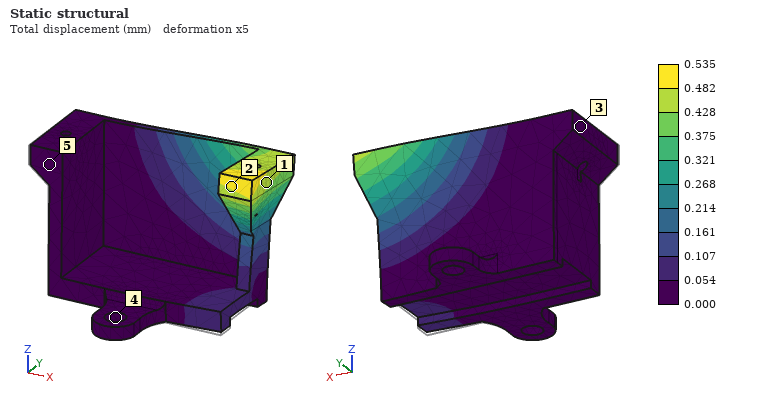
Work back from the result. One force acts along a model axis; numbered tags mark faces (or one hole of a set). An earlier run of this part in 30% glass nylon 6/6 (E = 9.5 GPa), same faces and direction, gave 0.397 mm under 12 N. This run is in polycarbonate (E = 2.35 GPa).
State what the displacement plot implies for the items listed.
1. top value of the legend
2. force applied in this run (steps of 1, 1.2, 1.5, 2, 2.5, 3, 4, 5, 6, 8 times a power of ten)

0.535 mm
4 N
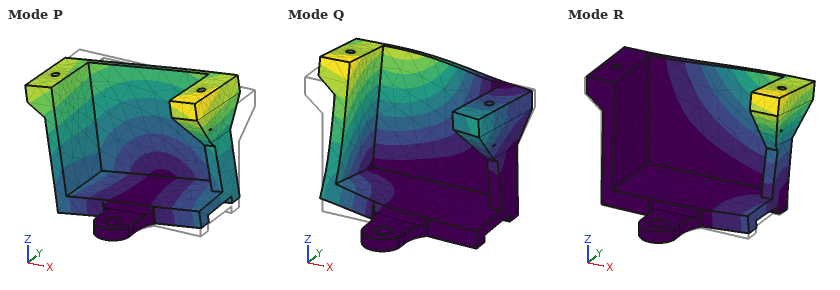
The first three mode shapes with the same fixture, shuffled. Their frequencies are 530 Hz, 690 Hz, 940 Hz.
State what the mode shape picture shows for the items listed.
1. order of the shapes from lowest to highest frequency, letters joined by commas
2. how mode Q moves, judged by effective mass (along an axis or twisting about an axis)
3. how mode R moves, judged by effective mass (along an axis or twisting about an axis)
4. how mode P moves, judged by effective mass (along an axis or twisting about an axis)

P, R, Q
along Y
along Y
along X
